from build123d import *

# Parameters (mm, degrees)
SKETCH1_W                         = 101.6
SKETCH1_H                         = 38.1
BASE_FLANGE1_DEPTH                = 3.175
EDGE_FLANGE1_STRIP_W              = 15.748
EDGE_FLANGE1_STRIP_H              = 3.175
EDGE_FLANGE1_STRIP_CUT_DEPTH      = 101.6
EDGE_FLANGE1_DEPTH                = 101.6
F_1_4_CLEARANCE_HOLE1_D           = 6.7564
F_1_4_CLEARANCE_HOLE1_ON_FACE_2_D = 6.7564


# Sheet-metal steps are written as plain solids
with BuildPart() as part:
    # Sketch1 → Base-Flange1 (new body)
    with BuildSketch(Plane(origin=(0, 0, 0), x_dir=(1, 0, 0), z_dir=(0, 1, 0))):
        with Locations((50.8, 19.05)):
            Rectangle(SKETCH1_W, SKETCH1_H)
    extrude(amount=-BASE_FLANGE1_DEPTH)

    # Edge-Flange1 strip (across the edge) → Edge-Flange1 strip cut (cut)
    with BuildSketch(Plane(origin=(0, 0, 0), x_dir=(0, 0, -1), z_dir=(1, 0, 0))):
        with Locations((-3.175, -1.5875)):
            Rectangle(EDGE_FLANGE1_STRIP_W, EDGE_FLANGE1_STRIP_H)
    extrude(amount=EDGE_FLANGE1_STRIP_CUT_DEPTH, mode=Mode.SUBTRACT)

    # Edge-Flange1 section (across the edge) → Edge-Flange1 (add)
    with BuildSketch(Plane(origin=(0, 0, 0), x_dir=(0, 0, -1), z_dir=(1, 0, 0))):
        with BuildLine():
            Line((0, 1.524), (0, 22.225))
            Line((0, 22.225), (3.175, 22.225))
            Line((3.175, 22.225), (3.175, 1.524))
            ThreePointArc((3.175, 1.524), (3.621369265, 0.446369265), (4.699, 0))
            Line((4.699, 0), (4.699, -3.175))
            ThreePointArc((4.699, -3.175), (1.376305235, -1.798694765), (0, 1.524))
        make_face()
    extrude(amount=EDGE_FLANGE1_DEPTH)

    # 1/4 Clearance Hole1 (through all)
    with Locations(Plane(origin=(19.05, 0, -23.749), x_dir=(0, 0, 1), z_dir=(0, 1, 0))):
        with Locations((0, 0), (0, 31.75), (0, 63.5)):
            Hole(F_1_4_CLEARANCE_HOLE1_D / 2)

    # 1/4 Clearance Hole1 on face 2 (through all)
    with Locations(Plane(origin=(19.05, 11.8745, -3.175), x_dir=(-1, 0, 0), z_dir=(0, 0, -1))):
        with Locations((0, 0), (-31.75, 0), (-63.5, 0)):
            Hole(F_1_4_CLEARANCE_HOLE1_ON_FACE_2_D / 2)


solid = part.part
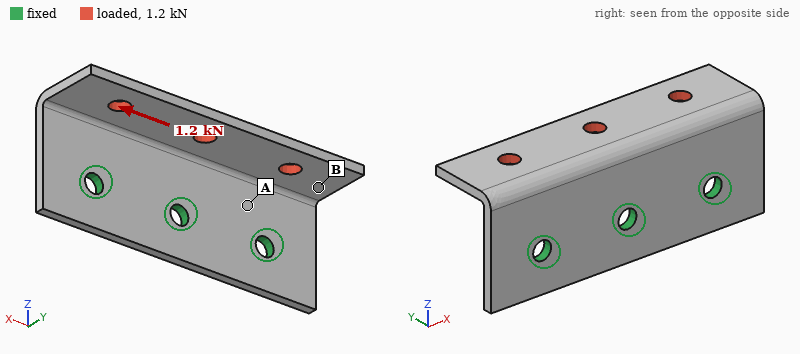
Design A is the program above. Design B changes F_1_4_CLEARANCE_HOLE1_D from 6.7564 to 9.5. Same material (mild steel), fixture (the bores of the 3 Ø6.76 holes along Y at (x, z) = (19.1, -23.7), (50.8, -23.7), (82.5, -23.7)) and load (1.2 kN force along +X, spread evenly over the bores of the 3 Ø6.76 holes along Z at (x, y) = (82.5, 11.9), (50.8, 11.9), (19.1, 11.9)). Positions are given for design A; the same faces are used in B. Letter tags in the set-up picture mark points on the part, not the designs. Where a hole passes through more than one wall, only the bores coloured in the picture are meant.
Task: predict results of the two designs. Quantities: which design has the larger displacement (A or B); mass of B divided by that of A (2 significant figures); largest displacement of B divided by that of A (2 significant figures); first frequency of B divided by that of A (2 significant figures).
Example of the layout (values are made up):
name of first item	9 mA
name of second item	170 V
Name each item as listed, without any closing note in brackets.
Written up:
which design has the larger displacement	A
mass of B divided by that of A	0.98
largest displacement of B divided by that of A	0.85
first frequency of B divided by that of A	1.1
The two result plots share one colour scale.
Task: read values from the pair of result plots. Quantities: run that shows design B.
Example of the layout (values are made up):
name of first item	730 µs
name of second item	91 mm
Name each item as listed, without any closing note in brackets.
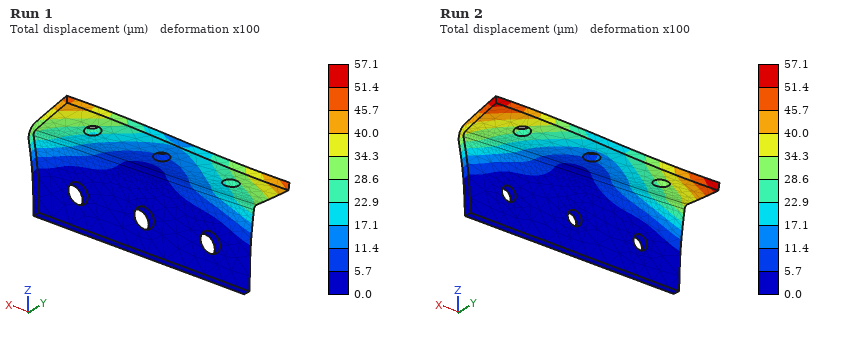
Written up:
run that shows design B	Run 1
